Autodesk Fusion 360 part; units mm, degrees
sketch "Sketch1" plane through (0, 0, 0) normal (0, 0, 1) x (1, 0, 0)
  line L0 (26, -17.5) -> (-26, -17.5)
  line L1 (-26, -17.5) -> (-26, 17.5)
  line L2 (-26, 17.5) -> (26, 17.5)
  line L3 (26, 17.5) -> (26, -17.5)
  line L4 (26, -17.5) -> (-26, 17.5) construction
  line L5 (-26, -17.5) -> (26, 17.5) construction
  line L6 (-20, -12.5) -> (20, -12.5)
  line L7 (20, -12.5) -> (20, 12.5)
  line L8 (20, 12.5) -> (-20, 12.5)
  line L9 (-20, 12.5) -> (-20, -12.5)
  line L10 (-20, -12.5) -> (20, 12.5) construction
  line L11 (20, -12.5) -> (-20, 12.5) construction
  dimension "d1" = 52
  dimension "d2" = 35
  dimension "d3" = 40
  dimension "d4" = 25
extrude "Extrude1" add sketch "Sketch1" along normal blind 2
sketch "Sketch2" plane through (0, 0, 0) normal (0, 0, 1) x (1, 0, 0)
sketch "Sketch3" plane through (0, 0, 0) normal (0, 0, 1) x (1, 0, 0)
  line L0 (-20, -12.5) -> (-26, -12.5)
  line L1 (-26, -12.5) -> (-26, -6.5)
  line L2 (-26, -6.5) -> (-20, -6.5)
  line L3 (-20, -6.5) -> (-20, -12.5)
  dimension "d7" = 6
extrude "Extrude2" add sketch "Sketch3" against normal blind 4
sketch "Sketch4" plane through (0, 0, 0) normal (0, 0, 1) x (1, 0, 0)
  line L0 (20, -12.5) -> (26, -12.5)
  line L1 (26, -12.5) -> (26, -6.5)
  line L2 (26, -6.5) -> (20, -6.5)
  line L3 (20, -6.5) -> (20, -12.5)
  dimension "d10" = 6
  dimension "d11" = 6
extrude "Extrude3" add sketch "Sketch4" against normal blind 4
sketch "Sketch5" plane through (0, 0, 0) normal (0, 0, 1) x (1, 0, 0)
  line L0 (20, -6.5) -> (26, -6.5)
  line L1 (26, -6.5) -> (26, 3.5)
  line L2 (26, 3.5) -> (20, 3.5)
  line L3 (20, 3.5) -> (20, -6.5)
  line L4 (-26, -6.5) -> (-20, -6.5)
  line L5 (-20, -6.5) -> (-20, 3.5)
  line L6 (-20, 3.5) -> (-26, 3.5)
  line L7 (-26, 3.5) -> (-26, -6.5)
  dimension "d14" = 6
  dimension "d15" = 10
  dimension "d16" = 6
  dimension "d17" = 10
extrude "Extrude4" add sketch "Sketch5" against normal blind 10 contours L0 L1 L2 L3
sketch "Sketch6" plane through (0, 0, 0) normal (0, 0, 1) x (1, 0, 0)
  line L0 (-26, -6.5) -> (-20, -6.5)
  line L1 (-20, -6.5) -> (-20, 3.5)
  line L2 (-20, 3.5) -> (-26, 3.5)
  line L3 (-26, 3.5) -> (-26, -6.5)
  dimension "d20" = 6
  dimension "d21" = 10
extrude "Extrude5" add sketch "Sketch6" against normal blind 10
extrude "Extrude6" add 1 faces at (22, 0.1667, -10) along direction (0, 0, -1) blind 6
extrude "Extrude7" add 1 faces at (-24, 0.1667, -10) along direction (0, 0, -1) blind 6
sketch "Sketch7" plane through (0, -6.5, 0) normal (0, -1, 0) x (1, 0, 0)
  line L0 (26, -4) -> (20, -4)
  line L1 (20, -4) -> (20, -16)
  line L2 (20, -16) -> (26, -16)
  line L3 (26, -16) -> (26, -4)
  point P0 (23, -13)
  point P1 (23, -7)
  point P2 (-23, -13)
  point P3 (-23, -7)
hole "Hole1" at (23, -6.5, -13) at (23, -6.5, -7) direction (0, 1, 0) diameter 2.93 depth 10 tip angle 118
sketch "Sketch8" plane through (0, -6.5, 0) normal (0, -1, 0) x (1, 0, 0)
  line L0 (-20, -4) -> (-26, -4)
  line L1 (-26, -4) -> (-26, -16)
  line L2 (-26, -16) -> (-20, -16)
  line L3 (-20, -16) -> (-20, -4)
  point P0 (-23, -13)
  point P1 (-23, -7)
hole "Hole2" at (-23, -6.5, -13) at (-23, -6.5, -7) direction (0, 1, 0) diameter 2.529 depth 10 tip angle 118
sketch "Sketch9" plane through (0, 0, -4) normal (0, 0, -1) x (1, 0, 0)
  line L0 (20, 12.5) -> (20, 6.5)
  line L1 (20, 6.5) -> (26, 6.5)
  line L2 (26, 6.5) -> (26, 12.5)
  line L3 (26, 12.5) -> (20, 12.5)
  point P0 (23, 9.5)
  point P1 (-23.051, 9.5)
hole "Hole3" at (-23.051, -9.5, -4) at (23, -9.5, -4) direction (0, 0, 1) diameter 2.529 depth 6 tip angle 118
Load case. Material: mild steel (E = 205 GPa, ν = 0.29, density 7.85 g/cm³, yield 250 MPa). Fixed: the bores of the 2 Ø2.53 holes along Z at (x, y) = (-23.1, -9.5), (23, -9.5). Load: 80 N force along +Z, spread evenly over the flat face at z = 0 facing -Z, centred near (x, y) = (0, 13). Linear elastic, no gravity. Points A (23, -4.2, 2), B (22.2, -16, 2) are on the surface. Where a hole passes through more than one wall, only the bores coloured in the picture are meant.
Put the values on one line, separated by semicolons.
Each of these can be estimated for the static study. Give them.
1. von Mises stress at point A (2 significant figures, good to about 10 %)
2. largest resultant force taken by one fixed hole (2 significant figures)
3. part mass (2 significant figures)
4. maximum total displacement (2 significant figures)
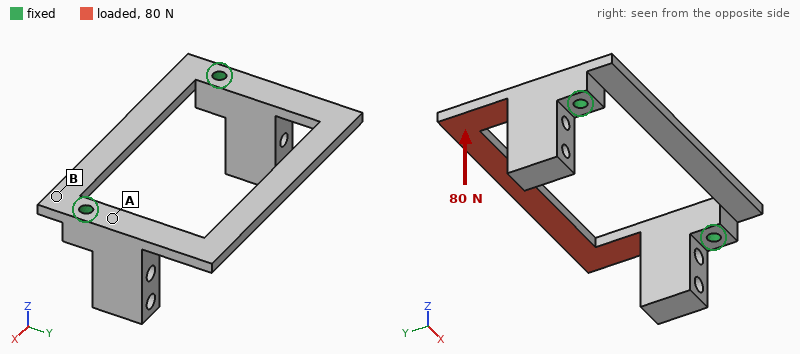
15 MPa; 40 N; 28 g; 71 µm
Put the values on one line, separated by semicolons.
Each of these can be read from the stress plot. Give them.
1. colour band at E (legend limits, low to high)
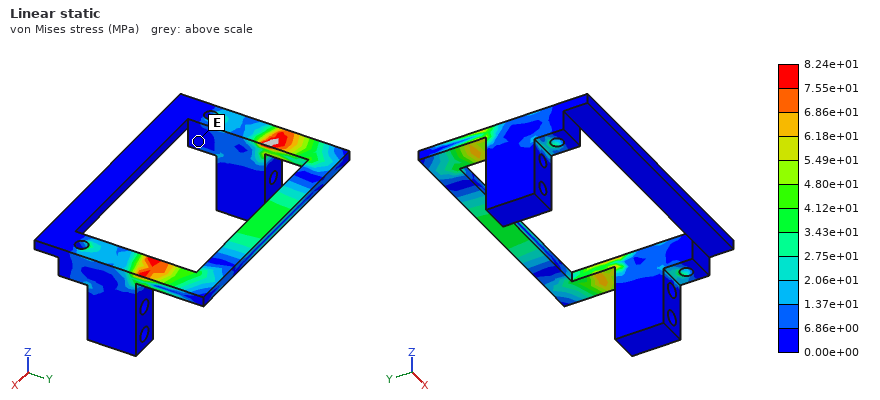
0.00e+00 to 6.86e+00 MPa
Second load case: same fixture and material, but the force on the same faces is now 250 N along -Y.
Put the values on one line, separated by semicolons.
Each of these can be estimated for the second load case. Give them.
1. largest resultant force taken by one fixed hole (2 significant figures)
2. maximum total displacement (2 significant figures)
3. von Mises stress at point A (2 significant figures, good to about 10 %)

130 N; 21 µm; 8.7 MPa
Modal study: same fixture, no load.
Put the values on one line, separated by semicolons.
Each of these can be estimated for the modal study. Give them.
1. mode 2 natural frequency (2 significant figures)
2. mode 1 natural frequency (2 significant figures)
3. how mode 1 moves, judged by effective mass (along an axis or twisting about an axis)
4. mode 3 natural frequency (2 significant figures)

5000 Hz; 2700 Hz; along Z; 5400 Hz
